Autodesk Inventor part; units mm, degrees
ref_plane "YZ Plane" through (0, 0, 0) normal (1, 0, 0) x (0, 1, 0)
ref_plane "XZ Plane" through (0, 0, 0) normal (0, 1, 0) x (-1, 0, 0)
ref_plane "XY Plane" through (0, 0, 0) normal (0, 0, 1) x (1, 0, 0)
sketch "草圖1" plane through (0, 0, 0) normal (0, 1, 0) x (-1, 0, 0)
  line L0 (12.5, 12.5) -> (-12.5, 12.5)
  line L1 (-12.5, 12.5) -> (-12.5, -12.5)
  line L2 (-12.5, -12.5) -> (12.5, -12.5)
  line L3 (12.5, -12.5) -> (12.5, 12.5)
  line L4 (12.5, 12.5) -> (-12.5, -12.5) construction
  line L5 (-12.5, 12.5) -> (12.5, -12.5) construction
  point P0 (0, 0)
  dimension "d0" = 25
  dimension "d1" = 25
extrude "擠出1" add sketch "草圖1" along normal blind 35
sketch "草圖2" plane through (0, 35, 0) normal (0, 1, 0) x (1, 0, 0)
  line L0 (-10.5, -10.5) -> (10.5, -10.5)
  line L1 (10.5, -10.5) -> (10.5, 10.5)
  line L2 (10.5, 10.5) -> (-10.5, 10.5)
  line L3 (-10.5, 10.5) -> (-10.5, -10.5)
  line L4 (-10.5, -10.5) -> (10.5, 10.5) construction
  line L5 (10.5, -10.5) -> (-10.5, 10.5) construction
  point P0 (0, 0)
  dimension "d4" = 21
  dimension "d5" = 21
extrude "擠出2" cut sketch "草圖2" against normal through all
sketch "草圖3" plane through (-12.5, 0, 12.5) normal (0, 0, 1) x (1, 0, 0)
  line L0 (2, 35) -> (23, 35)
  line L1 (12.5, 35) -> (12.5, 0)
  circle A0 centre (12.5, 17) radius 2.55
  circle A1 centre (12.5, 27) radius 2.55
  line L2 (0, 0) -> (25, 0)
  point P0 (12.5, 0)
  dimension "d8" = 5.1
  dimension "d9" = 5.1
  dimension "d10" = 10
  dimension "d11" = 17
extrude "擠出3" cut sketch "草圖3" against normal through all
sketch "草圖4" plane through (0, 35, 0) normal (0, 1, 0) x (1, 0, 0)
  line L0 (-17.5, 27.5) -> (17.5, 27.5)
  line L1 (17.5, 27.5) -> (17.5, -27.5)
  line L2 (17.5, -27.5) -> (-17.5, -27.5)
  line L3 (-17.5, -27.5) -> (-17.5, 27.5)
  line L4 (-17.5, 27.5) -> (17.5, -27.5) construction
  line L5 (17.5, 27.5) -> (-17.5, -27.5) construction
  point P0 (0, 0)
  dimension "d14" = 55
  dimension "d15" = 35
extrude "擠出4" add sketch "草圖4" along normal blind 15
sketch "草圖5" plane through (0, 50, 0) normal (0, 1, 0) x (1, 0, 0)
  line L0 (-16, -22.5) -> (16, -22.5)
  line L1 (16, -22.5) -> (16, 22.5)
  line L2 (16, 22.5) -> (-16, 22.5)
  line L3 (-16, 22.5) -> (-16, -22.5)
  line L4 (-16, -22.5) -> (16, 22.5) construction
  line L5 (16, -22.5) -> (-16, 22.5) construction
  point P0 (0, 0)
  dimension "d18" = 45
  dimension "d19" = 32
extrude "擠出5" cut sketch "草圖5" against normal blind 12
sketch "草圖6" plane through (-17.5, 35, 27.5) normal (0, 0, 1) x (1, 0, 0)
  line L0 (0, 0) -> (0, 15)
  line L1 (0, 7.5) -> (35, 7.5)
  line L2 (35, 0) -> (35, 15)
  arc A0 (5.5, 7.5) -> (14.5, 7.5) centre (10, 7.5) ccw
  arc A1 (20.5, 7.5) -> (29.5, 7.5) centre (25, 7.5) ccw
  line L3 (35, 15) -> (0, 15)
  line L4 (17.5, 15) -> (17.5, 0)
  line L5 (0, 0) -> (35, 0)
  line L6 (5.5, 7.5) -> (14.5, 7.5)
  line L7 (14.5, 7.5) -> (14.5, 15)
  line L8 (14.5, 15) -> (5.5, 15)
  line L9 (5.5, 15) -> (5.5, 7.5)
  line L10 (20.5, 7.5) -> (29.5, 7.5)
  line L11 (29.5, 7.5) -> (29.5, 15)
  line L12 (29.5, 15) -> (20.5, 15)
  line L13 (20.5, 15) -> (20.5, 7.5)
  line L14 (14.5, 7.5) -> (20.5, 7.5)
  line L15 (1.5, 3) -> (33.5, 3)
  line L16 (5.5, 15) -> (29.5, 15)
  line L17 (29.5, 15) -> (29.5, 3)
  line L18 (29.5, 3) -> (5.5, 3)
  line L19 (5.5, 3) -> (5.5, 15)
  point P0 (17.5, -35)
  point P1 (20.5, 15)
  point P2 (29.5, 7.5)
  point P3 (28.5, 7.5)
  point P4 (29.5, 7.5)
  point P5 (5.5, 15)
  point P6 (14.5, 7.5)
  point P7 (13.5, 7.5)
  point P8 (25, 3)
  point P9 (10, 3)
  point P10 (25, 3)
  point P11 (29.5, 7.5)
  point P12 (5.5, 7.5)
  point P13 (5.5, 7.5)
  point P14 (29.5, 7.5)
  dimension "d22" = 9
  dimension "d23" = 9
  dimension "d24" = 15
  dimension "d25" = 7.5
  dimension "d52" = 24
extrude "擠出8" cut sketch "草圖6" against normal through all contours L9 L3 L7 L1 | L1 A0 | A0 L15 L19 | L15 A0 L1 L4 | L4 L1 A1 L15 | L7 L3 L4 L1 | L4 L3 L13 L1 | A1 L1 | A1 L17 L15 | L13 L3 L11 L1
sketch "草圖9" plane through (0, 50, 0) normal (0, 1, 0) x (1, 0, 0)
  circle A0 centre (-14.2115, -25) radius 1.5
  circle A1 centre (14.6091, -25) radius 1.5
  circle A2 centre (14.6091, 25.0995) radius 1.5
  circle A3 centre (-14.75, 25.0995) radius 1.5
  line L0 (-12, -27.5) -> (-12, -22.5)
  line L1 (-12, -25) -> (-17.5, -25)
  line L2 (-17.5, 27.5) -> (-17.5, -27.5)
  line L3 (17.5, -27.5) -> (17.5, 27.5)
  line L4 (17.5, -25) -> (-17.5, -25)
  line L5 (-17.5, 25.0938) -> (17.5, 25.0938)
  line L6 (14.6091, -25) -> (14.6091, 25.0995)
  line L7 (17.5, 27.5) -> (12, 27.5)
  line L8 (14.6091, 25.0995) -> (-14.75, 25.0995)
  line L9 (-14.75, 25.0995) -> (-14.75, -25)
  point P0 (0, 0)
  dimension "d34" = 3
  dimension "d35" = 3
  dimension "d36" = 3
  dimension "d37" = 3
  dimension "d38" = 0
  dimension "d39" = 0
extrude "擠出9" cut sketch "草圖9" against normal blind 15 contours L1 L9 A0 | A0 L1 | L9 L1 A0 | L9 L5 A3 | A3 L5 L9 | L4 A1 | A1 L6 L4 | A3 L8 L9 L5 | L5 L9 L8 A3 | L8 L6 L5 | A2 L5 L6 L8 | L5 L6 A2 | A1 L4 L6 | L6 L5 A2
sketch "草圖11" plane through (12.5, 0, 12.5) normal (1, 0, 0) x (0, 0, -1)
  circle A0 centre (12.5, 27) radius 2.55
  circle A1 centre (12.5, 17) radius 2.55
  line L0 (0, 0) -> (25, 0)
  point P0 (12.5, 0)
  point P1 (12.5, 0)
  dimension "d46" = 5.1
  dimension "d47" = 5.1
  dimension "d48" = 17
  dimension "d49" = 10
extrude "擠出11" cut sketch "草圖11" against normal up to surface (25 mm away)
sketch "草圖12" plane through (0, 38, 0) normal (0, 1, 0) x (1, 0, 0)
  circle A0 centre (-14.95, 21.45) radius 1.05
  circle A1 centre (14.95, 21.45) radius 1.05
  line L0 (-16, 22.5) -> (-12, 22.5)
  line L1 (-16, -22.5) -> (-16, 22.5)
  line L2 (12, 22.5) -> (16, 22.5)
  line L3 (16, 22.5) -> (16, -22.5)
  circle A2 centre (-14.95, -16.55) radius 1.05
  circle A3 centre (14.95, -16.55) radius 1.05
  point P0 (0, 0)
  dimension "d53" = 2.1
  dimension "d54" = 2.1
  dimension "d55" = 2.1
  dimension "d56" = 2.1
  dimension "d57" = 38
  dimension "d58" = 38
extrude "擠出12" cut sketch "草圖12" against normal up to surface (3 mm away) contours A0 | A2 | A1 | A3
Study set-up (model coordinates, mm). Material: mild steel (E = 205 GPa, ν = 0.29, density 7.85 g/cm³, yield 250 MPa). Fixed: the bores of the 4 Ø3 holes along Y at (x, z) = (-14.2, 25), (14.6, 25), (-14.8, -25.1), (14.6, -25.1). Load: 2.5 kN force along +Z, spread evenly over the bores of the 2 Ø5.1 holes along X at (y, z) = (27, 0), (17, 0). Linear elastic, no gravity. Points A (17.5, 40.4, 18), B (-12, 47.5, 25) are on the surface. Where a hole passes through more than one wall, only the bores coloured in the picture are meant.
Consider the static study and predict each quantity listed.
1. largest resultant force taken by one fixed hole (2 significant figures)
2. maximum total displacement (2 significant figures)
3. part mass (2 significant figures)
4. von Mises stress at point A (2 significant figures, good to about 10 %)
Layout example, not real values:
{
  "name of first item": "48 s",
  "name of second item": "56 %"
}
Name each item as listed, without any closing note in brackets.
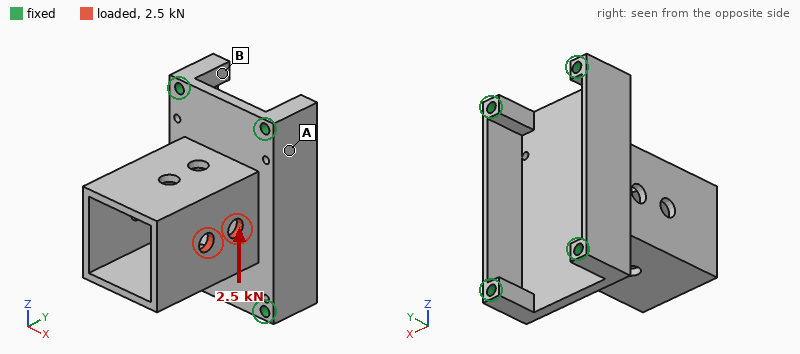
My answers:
{
  "largest resultant force taken by one fixed hole": "1.2 kN",
  "maximum total displacement": "53 µm",
  "part mass": "110 g",
  "von Mises stress at point A": "45 MPa"
}
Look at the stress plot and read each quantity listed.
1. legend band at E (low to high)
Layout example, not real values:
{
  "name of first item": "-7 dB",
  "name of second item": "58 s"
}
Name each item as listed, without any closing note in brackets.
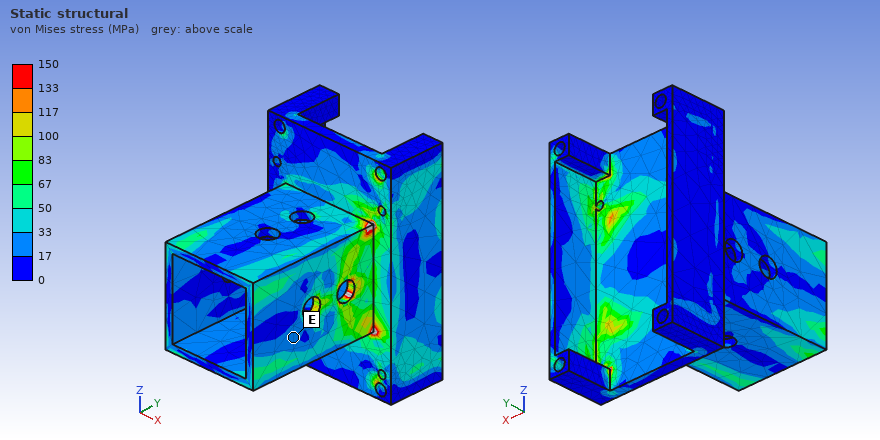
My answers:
{
  "legend band at E": "17 to 33 MPa"
}
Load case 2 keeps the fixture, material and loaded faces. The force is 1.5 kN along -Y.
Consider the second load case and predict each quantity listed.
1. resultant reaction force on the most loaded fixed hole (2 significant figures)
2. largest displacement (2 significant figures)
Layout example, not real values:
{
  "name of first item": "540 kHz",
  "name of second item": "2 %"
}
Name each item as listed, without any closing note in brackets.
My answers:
{
  "resultant reaction force on the most loaded fixed hole": "680 N",
  "largest displacement": "19 µm"
}
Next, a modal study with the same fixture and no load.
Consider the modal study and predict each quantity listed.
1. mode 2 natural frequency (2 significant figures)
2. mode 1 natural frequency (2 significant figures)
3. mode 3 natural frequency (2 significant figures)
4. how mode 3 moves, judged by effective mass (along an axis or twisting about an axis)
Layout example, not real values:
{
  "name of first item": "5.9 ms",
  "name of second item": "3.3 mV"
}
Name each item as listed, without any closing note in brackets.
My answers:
{
  "mode 2 natural frequency": "5700 Hz",
  "mode 1 natural frequency": "5600 Hz",
  "mode 3 natural frequency": "7600 Hz",
  "how mode 3 moves, judged by effective mass": "along Y"
}
